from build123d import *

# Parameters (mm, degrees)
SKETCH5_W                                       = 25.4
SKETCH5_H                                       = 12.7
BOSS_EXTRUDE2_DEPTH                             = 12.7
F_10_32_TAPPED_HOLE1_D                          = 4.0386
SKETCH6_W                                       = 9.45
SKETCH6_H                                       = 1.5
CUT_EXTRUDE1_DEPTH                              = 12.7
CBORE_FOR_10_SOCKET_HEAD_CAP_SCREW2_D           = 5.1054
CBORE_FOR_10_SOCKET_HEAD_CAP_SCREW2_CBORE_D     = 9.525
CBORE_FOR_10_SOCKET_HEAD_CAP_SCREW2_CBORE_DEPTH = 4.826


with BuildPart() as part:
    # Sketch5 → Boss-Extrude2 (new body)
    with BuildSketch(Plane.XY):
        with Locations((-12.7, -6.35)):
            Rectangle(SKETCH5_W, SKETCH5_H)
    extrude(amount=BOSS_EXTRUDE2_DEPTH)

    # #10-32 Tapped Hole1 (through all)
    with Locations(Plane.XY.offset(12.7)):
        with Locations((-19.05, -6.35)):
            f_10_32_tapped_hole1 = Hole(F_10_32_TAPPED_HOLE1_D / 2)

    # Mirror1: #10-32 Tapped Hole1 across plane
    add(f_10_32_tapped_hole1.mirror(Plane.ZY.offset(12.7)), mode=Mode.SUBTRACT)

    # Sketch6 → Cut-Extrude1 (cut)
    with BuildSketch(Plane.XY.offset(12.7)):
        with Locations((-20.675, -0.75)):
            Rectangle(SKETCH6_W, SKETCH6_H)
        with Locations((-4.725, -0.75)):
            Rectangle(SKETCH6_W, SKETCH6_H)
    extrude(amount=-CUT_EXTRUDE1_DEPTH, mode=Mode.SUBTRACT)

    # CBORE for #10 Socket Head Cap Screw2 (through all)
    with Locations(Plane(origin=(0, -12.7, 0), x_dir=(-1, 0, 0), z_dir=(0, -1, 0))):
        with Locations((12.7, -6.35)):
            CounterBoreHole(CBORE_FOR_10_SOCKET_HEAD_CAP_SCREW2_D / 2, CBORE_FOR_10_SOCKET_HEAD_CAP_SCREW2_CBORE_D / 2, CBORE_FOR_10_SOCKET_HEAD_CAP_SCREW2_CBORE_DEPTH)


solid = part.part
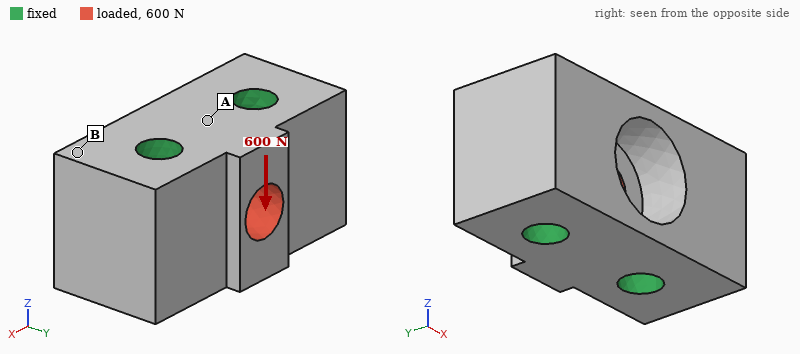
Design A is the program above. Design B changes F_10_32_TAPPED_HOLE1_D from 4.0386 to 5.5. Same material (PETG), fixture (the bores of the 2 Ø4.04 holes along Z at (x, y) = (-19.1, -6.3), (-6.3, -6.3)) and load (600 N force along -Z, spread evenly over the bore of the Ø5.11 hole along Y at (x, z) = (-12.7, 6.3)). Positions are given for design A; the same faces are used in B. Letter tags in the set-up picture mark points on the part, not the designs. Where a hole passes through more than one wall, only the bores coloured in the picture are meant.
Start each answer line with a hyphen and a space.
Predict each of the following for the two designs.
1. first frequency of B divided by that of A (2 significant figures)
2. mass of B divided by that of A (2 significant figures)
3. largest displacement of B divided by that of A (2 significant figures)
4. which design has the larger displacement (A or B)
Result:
- 1.3
- 0.90
- 0.84
- A
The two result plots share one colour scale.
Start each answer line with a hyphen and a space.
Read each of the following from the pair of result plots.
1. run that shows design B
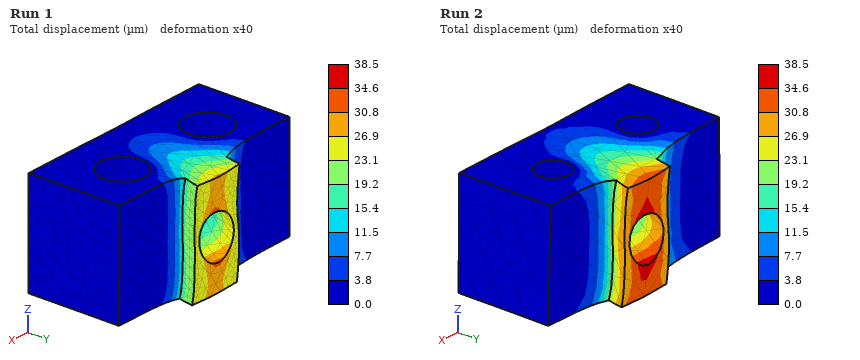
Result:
- Run 1
